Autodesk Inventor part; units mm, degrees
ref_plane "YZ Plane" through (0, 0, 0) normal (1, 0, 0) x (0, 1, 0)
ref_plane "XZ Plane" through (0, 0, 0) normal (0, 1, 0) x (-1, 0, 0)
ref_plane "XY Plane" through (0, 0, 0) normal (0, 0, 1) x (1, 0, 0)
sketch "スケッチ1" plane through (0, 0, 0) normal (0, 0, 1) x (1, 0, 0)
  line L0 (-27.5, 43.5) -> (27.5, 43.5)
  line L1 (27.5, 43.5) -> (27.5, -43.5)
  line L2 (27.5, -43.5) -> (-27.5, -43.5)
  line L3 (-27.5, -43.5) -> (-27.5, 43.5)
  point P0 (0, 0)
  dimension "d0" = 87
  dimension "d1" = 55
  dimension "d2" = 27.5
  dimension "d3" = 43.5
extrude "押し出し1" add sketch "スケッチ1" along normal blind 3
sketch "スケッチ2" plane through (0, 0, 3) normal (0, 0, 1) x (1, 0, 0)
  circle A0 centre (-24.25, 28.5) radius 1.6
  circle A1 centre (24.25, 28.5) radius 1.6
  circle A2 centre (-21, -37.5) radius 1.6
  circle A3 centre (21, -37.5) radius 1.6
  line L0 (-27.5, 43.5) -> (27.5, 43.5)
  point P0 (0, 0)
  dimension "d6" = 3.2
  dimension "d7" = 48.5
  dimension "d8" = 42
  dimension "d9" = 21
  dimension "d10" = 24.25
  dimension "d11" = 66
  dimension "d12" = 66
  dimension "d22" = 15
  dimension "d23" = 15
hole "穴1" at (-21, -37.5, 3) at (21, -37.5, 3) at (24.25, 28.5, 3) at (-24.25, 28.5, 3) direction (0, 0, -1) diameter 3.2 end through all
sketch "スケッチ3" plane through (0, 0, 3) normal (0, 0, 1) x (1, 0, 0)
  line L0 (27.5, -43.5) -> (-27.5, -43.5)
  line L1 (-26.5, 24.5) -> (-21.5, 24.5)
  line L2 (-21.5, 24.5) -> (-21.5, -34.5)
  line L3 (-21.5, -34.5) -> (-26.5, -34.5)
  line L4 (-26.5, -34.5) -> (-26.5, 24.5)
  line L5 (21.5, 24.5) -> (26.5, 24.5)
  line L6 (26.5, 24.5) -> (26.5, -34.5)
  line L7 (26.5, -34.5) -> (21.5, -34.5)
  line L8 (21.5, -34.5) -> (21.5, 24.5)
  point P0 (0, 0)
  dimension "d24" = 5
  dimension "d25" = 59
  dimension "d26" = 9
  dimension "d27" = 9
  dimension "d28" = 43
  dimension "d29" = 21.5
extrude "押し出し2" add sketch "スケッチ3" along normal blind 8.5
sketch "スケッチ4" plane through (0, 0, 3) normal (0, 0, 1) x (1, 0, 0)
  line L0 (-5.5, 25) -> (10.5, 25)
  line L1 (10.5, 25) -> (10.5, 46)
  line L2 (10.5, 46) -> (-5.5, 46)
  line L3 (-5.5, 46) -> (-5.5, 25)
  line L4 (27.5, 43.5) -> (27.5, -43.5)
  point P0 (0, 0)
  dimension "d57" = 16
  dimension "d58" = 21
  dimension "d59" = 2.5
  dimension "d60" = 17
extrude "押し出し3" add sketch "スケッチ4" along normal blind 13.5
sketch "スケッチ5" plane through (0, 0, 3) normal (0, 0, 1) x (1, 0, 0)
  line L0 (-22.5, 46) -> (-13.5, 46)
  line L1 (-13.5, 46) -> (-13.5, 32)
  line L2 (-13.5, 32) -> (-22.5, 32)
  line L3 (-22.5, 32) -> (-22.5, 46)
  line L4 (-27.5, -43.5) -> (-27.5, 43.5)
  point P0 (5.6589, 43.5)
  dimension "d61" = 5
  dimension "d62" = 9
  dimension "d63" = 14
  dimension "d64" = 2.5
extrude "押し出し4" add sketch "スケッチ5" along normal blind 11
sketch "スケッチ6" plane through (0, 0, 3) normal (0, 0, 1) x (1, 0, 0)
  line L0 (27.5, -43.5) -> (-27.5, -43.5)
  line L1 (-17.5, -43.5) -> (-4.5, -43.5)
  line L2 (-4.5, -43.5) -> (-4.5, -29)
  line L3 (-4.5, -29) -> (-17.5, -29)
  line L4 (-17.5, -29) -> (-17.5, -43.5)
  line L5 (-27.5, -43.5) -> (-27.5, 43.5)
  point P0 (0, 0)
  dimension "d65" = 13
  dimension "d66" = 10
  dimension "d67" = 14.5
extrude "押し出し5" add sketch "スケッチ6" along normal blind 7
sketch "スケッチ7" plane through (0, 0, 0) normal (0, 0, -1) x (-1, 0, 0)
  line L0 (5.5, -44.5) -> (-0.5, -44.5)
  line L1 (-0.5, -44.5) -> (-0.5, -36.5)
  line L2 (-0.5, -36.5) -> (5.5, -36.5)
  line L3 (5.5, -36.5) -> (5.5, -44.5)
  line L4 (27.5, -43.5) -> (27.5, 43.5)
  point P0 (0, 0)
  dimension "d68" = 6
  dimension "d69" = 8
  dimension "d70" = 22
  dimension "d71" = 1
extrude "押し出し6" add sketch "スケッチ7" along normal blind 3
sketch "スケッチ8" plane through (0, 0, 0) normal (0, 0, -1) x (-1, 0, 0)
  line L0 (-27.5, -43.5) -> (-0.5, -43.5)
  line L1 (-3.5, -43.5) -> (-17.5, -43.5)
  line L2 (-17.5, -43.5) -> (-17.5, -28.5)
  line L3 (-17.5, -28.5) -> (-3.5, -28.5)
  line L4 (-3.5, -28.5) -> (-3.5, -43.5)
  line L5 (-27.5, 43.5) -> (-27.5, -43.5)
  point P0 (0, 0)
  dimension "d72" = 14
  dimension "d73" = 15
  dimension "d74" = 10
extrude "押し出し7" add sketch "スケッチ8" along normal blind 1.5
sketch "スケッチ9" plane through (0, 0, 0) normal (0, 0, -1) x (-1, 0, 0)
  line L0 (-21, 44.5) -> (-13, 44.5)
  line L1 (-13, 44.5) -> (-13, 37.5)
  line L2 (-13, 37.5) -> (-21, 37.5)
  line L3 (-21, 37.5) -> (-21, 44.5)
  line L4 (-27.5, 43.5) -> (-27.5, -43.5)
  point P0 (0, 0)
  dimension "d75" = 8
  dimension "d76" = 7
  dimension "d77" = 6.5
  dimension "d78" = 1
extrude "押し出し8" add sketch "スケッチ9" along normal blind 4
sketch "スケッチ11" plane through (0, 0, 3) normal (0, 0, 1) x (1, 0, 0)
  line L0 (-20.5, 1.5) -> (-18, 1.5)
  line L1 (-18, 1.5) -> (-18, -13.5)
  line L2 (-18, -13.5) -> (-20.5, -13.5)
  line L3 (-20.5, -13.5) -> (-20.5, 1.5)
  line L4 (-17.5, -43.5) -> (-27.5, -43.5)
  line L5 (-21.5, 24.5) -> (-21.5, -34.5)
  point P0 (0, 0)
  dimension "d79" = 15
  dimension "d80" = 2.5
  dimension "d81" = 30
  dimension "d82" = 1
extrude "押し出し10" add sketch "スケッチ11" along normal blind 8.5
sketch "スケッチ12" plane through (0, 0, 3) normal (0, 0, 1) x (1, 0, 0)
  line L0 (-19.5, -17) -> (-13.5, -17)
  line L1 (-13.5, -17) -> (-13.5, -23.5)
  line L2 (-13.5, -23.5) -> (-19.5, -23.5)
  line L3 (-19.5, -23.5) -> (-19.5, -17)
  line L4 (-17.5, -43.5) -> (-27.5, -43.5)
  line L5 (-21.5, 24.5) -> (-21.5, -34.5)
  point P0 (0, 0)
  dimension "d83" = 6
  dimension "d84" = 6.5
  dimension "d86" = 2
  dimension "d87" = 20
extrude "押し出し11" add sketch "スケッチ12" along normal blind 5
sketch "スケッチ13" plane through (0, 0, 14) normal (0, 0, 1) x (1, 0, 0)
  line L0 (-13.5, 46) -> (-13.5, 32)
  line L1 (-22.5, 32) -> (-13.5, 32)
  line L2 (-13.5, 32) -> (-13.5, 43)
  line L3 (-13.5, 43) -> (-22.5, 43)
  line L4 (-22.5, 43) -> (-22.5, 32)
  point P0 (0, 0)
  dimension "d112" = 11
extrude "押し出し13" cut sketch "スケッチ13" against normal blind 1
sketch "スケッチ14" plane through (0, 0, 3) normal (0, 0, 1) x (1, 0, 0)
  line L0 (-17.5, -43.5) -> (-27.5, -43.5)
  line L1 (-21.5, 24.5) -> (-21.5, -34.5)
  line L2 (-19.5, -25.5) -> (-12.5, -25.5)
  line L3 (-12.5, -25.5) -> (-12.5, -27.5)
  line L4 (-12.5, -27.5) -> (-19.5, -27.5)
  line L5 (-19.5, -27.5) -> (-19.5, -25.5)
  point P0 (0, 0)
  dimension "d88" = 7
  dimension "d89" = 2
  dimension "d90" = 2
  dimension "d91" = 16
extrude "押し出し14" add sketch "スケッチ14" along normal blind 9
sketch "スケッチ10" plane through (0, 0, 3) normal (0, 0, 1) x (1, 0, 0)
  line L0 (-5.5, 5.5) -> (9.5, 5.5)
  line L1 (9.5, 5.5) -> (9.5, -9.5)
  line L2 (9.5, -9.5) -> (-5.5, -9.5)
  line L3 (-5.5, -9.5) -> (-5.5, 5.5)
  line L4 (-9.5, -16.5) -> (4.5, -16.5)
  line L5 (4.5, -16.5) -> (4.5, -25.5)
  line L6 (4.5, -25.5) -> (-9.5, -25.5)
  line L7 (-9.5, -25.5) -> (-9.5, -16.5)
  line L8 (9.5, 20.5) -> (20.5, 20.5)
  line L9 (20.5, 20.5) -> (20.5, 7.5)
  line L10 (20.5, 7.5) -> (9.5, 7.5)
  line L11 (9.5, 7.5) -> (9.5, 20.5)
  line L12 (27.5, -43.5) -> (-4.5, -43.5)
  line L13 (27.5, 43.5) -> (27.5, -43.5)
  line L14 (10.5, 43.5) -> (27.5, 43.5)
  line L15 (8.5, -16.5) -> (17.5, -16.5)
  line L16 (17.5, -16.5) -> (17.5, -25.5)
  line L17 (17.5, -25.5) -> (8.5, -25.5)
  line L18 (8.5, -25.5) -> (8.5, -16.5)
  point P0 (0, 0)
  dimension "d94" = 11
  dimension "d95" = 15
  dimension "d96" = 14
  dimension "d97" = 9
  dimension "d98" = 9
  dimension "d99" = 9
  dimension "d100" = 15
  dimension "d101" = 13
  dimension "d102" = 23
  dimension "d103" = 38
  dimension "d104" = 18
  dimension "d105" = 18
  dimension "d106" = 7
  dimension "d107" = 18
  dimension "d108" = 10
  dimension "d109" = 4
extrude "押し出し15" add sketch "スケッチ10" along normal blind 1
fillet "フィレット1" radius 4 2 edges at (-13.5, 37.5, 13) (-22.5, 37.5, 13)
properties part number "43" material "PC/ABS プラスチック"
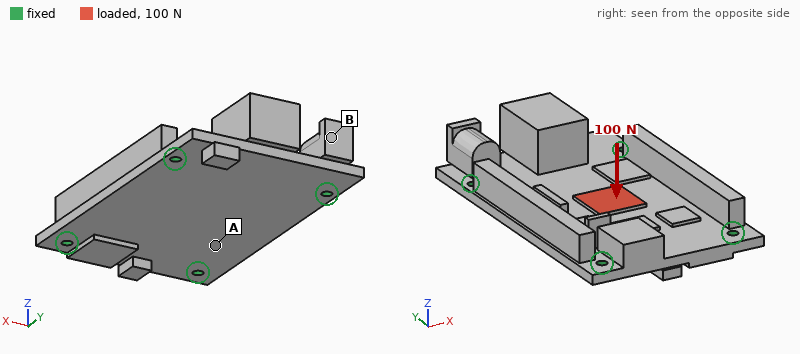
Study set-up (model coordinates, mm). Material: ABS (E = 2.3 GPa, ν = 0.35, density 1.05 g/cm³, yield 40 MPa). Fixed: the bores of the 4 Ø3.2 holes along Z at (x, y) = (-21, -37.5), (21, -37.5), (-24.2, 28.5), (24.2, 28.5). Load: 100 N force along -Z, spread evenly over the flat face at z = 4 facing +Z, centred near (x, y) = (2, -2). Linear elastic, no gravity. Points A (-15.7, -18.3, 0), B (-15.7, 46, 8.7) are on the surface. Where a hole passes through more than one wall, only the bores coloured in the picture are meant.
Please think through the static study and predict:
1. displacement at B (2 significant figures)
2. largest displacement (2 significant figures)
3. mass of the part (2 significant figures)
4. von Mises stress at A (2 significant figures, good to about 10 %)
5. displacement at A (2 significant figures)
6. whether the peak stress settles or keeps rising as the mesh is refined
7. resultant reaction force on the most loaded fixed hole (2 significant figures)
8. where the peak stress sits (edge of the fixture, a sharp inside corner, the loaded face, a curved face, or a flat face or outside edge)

0.067 mm
0.32 mm
30 g
2.1 MPa
0.12 mm
keeps rising
43 N
edge of the fixture
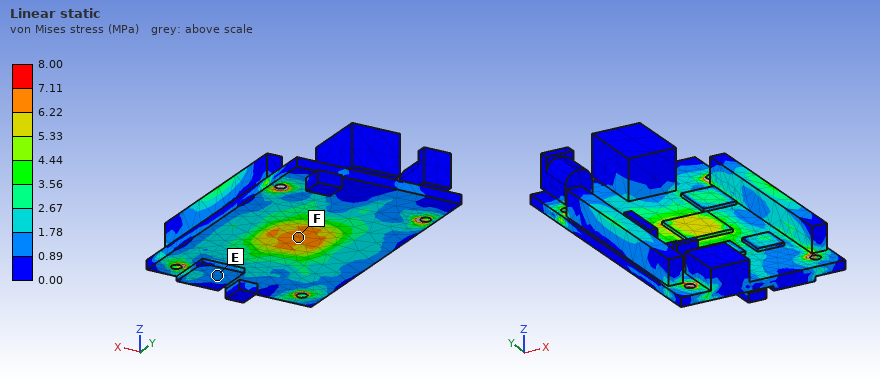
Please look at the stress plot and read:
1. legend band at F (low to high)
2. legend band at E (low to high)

6.22 to 7.11 MPa
0.89 to 1.78 MPa
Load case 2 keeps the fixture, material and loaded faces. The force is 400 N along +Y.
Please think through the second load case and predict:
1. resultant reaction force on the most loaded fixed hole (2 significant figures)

110 N
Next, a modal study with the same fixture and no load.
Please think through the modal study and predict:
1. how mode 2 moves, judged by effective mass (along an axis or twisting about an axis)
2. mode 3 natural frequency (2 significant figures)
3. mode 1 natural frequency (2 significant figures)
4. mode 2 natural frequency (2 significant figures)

along Z
1900 Hz
820 Hz
1300 Hz
